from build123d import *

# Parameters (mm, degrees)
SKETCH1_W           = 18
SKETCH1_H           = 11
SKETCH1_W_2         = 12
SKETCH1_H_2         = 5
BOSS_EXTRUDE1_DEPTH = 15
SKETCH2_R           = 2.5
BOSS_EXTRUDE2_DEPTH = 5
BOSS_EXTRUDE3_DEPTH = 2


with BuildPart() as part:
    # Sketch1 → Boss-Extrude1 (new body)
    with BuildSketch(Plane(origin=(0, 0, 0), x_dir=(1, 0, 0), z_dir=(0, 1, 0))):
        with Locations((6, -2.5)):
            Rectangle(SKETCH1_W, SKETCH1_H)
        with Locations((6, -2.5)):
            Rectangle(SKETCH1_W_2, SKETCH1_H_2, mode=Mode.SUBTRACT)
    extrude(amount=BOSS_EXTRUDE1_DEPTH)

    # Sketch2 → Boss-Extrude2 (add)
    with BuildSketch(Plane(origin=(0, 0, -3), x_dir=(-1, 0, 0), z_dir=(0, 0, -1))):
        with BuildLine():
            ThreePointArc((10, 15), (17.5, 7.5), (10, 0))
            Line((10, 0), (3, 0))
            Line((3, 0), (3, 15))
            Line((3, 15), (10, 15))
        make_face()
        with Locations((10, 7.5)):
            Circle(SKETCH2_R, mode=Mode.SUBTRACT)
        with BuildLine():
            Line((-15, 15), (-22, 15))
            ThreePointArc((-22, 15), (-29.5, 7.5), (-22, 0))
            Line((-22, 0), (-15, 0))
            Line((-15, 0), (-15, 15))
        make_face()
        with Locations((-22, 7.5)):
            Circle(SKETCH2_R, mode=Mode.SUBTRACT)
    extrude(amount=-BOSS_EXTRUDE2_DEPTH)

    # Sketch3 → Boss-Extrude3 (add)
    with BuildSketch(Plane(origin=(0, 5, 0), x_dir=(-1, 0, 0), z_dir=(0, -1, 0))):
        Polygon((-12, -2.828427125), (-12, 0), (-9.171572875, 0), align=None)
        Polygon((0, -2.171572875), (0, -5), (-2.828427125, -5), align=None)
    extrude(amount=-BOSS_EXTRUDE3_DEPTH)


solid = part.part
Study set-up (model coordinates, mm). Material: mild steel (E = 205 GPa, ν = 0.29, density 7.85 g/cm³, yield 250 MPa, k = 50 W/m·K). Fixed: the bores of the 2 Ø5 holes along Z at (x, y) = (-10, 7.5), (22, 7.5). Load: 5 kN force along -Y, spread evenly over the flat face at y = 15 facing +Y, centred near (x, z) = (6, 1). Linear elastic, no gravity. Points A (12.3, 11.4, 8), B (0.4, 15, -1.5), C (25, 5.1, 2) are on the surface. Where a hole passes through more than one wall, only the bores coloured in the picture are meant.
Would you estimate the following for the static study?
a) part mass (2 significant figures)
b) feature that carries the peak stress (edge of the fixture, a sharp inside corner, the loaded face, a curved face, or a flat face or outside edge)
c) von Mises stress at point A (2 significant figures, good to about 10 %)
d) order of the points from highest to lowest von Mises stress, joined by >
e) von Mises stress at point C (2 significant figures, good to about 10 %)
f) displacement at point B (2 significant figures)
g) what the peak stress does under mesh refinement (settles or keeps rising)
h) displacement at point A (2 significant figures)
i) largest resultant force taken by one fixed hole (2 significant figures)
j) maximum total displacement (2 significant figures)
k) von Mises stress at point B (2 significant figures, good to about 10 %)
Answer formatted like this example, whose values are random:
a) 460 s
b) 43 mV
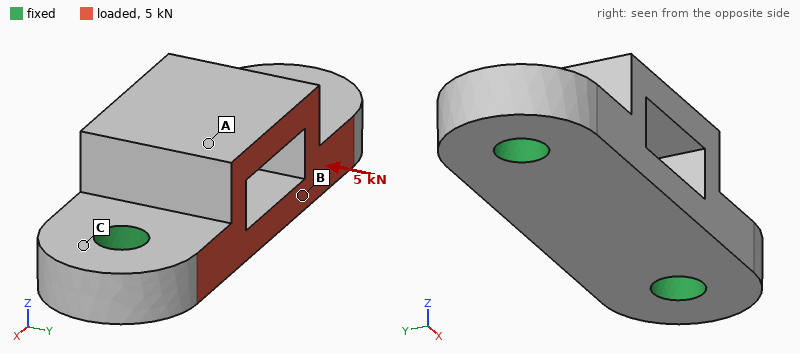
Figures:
a) 30 g
b) edge of the fixture
c) 32 MPa
d) B > A > C
e) 21 MPa
f) 7.4 µm
g) keeps rising
h) 13 µm
i) 2.5 kN
j) 15 µm
k) 58 MPa
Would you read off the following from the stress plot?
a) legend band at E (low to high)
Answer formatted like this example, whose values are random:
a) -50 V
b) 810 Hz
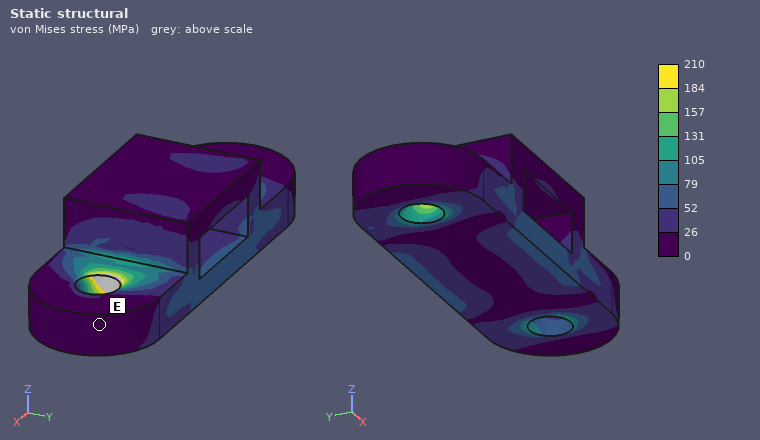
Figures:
a) 0 to 26 MPa
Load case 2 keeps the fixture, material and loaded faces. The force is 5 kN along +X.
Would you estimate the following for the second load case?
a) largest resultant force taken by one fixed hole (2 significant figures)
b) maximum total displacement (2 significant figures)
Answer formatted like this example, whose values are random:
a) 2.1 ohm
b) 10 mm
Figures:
a) 2.7 kN
b) 12 µm
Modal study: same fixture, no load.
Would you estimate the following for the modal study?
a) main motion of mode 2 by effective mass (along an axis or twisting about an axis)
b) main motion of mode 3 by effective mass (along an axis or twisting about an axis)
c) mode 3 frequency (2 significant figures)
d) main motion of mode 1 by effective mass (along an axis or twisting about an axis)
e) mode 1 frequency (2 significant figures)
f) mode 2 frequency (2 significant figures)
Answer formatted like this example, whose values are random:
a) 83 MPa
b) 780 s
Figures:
a) along Z
b) along X
c) 34 kHz
d) along Y
e) 20 kHz
f) 26 kHz
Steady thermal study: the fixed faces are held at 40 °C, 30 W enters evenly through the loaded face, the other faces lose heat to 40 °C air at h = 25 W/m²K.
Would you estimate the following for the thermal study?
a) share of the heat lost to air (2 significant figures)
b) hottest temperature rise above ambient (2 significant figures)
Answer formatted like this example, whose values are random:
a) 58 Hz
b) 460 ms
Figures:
a) 3.9 %
b) 51 K
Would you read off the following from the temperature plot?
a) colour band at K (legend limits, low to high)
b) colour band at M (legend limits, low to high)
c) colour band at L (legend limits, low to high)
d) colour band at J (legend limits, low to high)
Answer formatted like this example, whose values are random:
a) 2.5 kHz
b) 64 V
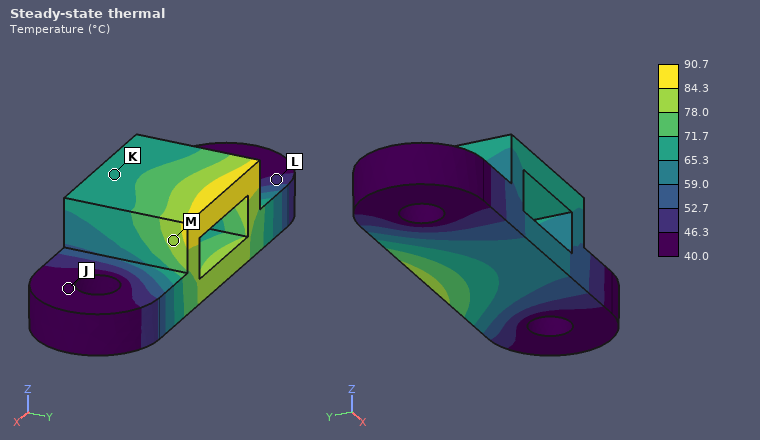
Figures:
a) 65.3 to 71.7 °C
b) 78.0 to 84.3 °C
c) 46.3 to 52.7 °C
d) 40.0 to 46.3 °C
